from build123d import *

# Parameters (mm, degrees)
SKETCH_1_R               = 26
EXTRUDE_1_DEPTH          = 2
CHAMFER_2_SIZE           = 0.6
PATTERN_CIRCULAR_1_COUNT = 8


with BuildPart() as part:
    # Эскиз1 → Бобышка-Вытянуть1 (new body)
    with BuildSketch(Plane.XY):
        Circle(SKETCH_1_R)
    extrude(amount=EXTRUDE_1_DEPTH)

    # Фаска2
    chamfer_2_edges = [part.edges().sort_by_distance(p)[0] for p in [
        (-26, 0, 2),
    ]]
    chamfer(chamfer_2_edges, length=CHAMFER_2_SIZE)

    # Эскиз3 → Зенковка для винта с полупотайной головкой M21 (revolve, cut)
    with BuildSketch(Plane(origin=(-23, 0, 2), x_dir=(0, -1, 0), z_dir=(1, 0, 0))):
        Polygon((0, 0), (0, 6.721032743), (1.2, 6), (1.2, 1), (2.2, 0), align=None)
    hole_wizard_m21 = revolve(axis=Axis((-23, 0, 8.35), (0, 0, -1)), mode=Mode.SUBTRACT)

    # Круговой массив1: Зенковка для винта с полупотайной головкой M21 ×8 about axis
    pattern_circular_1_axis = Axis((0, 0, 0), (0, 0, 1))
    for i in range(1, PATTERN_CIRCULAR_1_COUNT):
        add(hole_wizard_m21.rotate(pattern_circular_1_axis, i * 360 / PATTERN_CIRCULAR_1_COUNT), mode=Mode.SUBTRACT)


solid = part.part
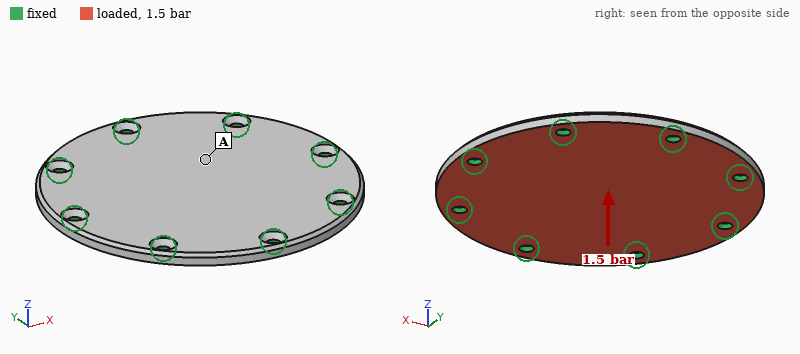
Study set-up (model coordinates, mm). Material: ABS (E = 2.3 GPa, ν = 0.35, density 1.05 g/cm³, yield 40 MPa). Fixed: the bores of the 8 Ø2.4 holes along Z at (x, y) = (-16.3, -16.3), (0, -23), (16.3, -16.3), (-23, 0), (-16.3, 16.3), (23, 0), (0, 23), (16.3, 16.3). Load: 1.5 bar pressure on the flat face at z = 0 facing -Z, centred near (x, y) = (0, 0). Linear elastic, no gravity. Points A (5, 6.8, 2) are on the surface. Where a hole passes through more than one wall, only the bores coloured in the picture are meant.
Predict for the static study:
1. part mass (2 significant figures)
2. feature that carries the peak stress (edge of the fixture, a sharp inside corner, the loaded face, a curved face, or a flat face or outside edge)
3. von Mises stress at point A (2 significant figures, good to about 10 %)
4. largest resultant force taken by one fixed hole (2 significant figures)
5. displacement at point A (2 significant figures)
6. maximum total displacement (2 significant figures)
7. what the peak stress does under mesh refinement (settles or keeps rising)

4.3 g
edge of the fixture
11 MPa
50 N
0.46 mm
0.57 mm
keeps rising
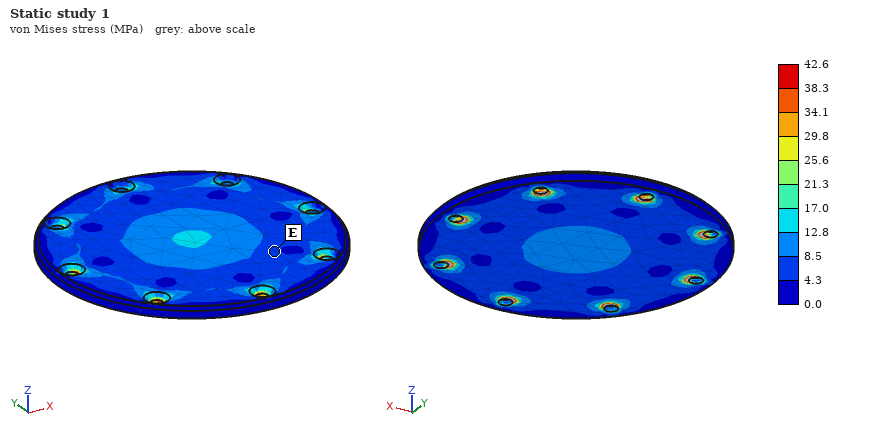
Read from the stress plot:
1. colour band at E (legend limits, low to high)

4.3 to 8.5 MPa
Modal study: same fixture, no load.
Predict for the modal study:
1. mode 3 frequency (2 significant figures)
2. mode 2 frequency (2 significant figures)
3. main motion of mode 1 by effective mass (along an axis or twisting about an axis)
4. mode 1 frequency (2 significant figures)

4600 Hz
4600 Hz
along Z
2200 Hz
